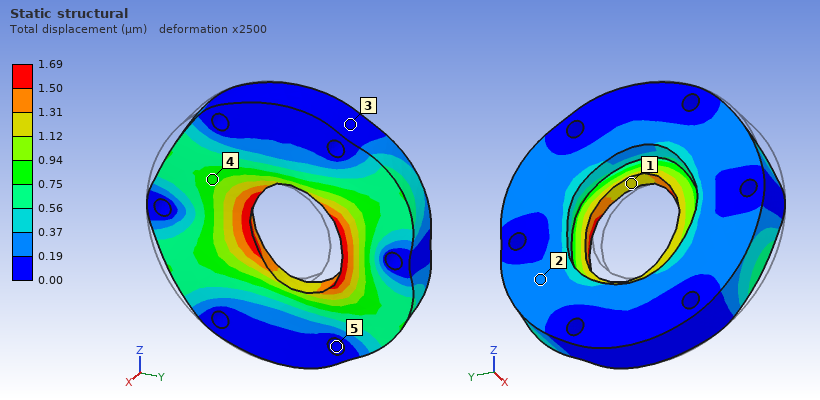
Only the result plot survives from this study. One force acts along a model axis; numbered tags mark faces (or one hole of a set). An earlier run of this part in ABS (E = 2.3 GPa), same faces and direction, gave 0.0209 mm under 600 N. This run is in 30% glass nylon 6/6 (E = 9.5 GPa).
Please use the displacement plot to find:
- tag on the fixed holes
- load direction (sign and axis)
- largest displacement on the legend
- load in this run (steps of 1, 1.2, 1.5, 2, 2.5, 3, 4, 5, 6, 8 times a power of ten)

5
+Y
1.69 µm
200 N
